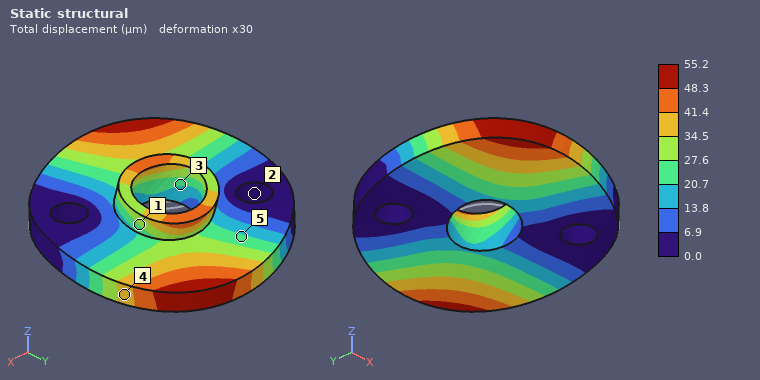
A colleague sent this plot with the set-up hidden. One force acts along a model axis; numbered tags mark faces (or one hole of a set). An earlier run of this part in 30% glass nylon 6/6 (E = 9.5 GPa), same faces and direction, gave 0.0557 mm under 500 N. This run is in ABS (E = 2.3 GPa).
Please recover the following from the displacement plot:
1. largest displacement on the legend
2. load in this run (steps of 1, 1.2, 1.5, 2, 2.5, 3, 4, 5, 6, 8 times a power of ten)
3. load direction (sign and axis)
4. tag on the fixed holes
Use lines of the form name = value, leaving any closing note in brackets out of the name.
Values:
largest displacement on the legend = 55.2 µm
load in this run = 120 N
load direction = +Y
tag on the fixed holes = 2
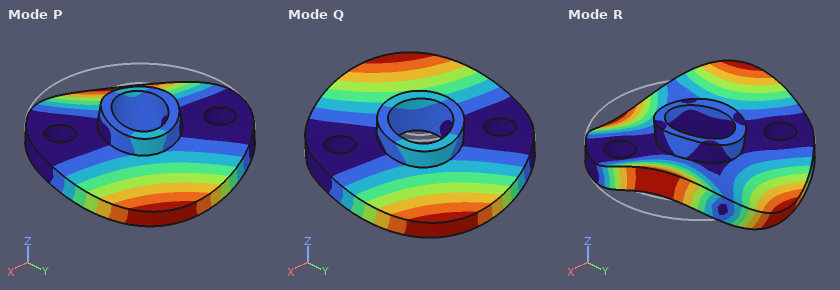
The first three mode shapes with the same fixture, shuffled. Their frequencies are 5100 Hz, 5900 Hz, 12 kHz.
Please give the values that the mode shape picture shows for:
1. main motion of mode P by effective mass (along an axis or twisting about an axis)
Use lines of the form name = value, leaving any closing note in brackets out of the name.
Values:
main motion of mode P by effective mass = along Z
